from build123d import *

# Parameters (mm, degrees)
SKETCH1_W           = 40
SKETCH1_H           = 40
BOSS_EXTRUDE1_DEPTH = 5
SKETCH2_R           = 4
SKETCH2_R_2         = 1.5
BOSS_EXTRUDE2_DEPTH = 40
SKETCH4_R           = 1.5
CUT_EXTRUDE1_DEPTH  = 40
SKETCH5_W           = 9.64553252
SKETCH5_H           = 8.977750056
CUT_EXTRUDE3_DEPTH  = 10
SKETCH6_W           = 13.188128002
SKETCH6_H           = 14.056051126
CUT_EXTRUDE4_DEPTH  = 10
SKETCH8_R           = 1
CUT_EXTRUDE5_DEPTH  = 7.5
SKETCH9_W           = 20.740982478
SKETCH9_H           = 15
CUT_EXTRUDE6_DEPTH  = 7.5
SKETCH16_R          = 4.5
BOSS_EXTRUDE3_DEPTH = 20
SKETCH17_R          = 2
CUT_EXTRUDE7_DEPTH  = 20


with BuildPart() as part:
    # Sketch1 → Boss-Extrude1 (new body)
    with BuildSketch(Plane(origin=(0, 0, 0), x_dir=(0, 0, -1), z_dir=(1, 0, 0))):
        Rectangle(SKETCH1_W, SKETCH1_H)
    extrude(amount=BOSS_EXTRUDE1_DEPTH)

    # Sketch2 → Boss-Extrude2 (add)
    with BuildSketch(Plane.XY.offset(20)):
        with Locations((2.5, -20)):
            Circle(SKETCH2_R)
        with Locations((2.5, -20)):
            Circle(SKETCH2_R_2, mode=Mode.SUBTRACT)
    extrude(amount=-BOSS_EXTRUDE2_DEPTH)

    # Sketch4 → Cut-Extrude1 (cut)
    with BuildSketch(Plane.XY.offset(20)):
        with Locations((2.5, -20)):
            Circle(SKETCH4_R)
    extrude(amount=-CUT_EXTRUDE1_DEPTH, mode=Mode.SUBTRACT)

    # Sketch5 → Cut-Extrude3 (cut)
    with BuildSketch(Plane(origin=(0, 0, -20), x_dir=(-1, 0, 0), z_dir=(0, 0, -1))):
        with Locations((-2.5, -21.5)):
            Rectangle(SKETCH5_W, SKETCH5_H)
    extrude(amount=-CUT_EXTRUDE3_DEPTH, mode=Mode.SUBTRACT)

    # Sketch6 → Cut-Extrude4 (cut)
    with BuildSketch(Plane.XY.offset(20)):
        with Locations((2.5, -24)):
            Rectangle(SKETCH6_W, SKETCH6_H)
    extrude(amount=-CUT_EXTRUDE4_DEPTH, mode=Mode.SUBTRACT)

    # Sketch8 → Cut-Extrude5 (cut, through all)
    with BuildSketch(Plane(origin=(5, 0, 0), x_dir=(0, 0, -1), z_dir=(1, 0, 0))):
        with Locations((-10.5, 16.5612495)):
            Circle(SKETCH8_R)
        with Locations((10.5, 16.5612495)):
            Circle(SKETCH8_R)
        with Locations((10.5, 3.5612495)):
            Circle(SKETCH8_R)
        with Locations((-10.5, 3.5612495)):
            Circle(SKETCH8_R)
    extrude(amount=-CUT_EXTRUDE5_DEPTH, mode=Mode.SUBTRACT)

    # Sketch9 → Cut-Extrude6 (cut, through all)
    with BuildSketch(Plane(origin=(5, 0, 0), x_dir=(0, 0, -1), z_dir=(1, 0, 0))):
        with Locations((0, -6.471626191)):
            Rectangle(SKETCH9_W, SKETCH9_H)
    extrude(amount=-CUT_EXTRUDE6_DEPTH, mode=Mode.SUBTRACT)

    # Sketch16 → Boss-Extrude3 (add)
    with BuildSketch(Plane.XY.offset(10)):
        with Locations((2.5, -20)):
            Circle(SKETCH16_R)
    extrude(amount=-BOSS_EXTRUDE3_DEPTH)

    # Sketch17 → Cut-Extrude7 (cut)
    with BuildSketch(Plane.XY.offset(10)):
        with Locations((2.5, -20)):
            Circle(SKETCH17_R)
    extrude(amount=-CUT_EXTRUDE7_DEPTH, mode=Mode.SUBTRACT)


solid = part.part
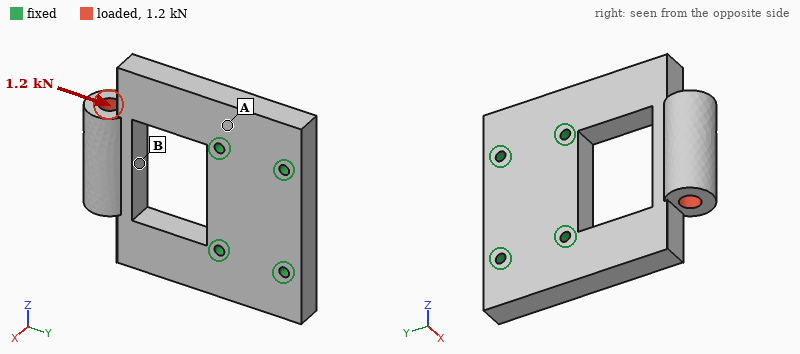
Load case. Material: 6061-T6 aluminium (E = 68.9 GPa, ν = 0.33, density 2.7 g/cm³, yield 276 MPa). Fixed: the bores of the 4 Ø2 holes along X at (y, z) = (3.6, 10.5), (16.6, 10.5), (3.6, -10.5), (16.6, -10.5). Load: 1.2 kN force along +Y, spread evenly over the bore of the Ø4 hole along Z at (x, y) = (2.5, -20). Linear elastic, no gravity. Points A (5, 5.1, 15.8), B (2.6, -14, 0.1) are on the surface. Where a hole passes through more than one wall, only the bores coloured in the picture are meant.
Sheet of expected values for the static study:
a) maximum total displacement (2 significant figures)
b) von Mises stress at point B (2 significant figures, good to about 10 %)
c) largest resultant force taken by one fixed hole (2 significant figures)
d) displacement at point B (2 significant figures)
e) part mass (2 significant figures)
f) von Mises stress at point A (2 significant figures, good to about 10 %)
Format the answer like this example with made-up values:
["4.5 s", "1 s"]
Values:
["21 µm", "31 MPa", "520 N", "21 µm", "18 g", "12 MPa"]
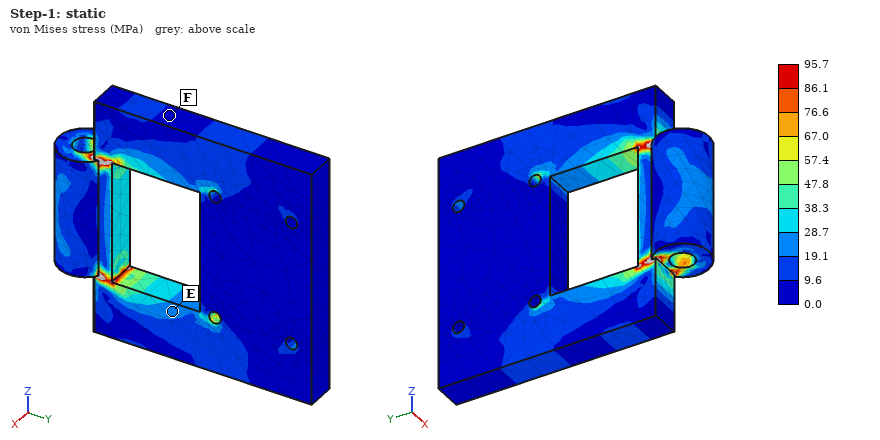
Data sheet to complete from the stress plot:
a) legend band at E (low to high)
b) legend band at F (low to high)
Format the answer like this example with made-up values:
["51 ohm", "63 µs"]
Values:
["19.1 to 28.7 MPa", "0.0 to 9.6 MPa"]
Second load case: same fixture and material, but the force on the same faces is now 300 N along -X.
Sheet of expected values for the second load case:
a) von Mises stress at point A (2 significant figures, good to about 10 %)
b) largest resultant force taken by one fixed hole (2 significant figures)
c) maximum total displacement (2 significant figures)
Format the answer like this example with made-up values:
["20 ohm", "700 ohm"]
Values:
["40 MPa", "270 N", "0.18 mm"]
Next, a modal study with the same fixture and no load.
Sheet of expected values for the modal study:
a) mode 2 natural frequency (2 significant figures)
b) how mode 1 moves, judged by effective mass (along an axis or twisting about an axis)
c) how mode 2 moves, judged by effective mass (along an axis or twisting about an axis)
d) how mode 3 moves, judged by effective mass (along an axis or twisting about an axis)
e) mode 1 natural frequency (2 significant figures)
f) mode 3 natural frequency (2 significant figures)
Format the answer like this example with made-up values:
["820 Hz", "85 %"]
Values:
["8800 Hz", "along X", "twisting about Y", "along Z", "3800 Hz", "9300 Hz"]
